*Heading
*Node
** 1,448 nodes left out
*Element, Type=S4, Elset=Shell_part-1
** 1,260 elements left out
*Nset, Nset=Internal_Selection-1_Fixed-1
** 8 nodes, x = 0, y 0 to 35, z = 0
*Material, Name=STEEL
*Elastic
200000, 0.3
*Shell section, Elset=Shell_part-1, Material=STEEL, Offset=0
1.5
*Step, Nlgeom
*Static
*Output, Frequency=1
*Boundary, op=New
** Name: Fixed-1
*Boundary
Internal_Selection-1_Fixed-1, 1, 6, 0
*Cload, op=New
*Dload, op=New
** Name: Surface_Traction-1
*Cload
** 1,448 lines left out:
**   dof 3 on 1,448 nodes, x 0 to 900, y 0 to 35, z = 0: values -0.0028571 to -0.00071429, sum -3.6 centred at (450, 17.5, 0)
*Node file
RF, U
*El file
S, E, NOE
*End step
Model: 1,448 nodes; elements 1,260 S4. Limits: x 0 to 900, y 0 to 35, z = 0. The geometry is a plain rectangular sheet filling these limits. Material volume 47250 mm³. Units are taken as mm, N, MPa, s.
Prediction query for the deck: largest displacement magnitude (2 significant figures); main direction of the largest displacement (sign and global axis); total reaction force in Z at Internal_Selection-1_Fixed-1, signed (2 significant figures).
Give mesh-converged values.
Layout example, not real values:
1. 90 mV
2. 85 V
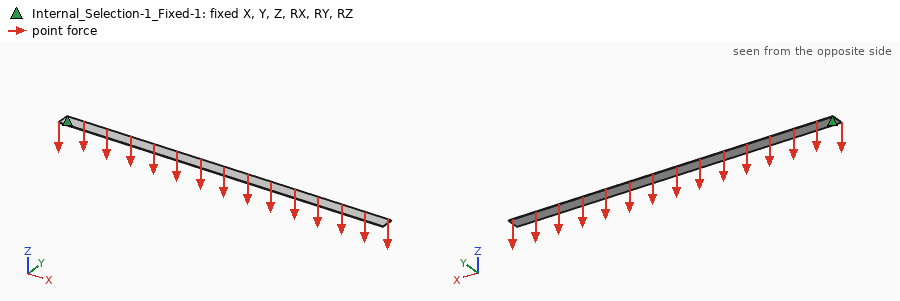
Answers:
1. 160 mm
2. -Z
3. 3.6 N
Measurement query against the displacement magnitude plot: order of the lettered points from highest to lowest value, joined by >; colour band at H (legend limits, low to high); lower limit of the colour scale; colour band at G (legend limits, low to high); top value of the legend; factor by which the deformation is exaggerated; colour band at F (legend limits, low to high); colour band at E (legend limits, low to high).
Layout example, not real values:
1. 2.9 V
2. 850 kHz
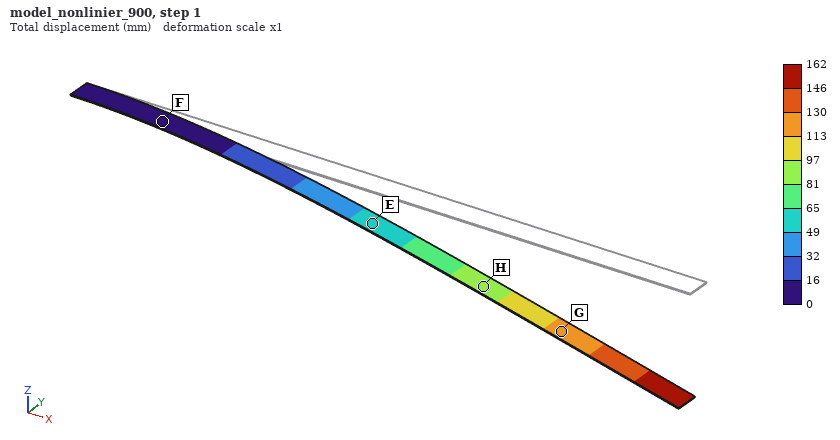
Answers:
1. G > H > E > F
2. 81 to 97 mm
3. 0 mm
4. 113 to 130 mm
5. 162 mm
6. 1
7. 0 to 16 mm
8. 49 to 65 mm
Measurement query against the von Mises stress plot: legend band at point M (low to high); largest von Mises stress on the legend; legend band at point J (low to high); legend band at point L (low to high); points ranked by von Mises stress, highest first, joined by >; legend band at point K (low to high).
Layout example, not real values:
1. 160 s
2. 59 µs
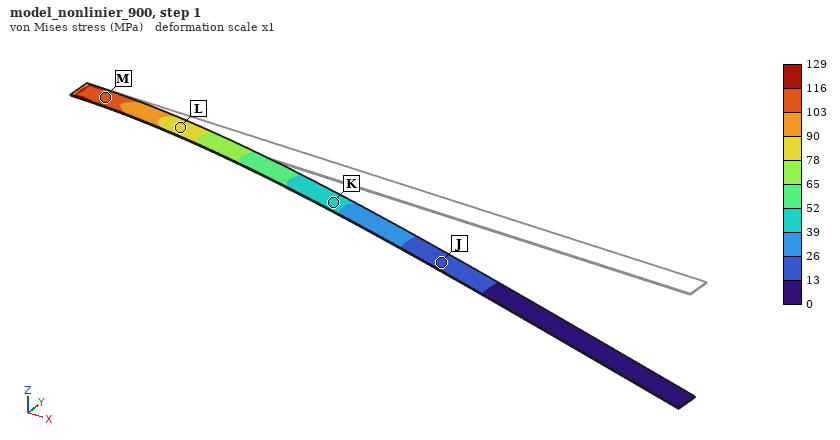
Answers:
1. 103 to 116 MPa
2. 129 MPa
3. 13 to 26 MPa
4. 78 to 90 MPa
5. M > L > K > J
6. 39 to 52 MPa
